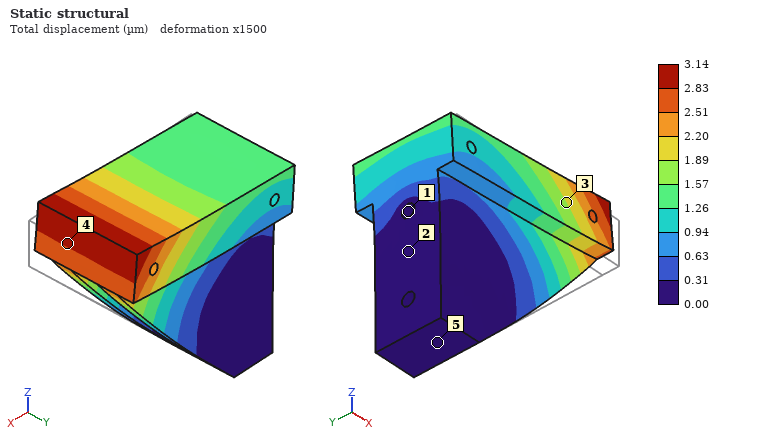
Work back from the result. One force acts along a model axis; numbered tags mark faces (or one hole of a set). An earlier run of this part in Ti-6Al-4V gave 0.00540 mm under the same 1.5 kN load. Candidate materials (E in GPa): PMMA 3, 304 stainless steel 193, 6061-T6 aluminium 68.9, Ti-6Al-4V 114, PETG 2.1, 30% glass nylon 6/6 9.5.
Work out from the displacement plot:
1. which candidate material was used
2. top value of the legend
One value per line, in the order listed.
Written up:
304 stainless steel
3.14 µm
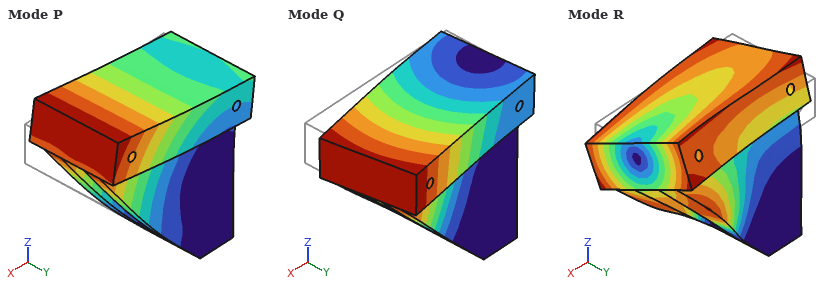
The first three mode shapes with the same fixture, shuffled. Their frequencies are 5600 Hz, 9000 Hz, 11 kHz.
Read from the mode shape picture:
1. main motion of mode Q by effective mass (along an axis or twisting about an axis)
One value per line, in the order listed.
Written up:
along Y
